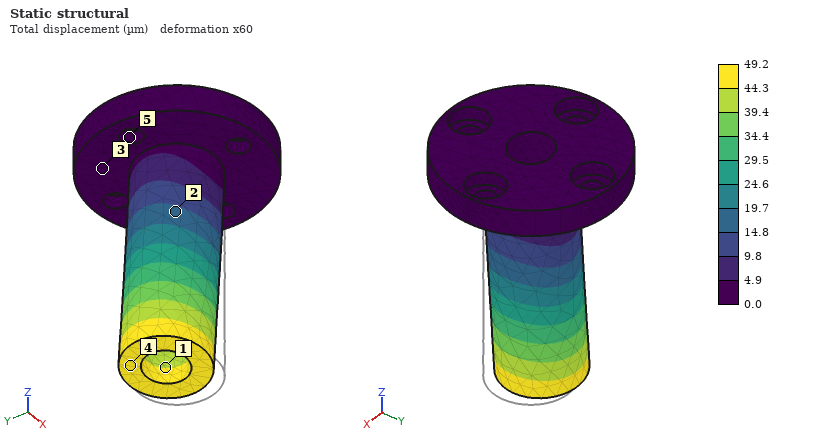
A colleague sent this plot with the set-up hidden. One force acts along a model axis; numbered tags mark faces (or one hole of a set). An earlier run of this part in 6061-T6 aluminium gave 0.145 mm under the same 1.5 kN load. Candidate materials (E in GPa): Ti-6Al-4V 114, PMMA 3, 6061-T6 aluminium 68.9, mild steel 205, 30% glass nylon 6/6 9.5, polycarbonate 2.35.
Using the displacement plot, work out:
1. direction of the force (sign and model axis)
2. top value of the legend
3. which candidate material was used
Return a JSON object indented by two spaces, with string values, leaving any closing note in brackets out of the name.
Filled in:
{
  "direction of the force": "-X",
  "top value of the legend": "49.2 µm",
  "which candidate material was used": "mild steel"
}
